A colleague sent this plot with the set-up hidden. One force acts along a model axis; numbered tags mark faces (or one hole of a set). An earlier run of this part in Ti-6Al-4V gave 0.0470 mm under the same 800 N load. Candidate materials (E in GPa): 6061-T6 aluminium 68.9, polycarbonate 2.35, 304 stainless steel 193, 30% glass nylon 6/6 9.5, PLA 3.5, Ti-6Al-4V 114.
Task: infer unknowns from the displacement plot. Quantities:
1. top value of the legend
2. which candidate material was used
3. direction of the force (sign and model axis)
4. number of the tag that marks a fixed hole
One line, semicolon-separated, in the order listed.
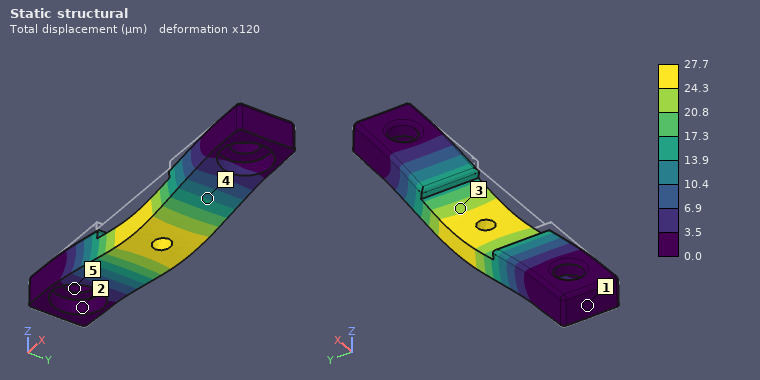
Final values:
27.7 µm; 304 stainless steel; -Z; 5
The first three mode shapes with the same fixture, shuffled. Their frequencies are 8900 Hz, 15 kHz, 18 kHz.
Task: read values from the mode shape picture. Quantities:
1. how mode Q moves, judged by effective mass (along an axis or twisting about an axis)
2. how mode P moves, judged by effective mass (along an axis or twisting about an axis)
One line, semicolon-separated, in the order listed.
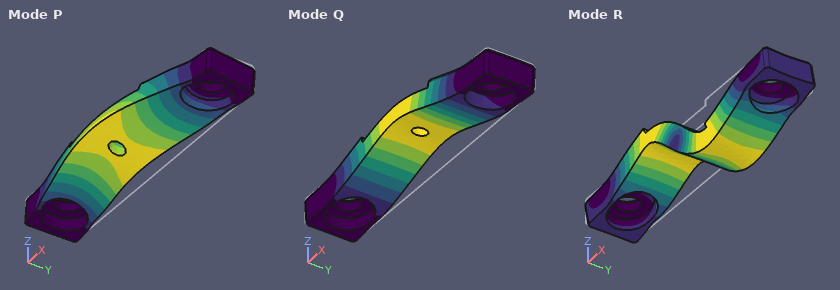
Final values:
along Z; along Y
